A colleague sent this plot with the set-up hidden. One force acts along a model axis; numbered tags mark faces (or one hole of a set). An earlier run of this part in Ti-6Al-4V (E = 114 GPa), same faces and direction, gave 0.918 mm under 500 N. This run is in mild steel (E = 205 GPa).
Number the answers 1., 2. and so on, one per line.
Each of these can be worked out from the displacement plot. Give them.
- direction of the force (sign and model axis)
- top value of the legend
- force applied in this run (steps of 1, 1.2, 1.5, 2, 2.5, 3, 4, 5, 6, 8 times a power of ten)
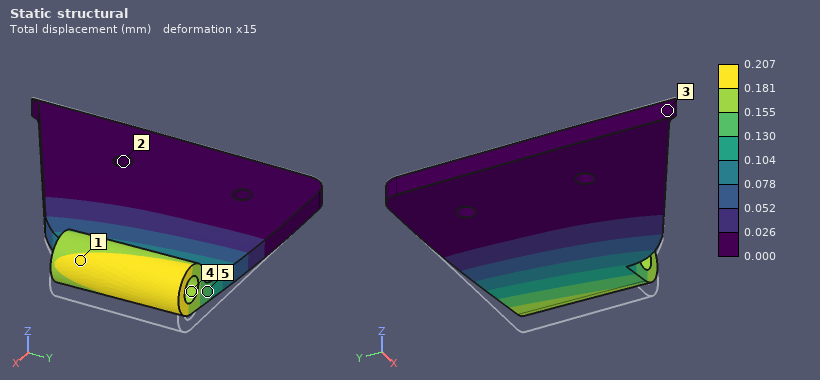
1. +Z
2. 0.207 mm
3. 200 N
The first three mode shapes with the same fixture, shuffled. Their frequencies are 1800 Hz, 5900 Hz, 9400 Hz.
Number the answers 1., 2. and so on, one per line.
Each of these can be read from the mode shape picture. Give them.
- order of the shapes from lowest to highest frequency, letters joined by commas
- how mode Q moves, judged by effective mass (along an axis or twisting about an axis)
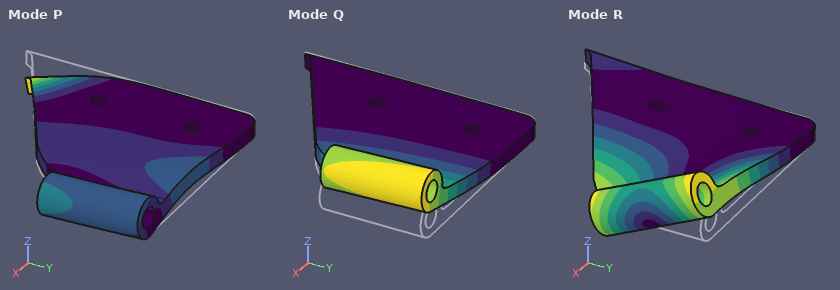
1. Q, R, P
2. along Z
